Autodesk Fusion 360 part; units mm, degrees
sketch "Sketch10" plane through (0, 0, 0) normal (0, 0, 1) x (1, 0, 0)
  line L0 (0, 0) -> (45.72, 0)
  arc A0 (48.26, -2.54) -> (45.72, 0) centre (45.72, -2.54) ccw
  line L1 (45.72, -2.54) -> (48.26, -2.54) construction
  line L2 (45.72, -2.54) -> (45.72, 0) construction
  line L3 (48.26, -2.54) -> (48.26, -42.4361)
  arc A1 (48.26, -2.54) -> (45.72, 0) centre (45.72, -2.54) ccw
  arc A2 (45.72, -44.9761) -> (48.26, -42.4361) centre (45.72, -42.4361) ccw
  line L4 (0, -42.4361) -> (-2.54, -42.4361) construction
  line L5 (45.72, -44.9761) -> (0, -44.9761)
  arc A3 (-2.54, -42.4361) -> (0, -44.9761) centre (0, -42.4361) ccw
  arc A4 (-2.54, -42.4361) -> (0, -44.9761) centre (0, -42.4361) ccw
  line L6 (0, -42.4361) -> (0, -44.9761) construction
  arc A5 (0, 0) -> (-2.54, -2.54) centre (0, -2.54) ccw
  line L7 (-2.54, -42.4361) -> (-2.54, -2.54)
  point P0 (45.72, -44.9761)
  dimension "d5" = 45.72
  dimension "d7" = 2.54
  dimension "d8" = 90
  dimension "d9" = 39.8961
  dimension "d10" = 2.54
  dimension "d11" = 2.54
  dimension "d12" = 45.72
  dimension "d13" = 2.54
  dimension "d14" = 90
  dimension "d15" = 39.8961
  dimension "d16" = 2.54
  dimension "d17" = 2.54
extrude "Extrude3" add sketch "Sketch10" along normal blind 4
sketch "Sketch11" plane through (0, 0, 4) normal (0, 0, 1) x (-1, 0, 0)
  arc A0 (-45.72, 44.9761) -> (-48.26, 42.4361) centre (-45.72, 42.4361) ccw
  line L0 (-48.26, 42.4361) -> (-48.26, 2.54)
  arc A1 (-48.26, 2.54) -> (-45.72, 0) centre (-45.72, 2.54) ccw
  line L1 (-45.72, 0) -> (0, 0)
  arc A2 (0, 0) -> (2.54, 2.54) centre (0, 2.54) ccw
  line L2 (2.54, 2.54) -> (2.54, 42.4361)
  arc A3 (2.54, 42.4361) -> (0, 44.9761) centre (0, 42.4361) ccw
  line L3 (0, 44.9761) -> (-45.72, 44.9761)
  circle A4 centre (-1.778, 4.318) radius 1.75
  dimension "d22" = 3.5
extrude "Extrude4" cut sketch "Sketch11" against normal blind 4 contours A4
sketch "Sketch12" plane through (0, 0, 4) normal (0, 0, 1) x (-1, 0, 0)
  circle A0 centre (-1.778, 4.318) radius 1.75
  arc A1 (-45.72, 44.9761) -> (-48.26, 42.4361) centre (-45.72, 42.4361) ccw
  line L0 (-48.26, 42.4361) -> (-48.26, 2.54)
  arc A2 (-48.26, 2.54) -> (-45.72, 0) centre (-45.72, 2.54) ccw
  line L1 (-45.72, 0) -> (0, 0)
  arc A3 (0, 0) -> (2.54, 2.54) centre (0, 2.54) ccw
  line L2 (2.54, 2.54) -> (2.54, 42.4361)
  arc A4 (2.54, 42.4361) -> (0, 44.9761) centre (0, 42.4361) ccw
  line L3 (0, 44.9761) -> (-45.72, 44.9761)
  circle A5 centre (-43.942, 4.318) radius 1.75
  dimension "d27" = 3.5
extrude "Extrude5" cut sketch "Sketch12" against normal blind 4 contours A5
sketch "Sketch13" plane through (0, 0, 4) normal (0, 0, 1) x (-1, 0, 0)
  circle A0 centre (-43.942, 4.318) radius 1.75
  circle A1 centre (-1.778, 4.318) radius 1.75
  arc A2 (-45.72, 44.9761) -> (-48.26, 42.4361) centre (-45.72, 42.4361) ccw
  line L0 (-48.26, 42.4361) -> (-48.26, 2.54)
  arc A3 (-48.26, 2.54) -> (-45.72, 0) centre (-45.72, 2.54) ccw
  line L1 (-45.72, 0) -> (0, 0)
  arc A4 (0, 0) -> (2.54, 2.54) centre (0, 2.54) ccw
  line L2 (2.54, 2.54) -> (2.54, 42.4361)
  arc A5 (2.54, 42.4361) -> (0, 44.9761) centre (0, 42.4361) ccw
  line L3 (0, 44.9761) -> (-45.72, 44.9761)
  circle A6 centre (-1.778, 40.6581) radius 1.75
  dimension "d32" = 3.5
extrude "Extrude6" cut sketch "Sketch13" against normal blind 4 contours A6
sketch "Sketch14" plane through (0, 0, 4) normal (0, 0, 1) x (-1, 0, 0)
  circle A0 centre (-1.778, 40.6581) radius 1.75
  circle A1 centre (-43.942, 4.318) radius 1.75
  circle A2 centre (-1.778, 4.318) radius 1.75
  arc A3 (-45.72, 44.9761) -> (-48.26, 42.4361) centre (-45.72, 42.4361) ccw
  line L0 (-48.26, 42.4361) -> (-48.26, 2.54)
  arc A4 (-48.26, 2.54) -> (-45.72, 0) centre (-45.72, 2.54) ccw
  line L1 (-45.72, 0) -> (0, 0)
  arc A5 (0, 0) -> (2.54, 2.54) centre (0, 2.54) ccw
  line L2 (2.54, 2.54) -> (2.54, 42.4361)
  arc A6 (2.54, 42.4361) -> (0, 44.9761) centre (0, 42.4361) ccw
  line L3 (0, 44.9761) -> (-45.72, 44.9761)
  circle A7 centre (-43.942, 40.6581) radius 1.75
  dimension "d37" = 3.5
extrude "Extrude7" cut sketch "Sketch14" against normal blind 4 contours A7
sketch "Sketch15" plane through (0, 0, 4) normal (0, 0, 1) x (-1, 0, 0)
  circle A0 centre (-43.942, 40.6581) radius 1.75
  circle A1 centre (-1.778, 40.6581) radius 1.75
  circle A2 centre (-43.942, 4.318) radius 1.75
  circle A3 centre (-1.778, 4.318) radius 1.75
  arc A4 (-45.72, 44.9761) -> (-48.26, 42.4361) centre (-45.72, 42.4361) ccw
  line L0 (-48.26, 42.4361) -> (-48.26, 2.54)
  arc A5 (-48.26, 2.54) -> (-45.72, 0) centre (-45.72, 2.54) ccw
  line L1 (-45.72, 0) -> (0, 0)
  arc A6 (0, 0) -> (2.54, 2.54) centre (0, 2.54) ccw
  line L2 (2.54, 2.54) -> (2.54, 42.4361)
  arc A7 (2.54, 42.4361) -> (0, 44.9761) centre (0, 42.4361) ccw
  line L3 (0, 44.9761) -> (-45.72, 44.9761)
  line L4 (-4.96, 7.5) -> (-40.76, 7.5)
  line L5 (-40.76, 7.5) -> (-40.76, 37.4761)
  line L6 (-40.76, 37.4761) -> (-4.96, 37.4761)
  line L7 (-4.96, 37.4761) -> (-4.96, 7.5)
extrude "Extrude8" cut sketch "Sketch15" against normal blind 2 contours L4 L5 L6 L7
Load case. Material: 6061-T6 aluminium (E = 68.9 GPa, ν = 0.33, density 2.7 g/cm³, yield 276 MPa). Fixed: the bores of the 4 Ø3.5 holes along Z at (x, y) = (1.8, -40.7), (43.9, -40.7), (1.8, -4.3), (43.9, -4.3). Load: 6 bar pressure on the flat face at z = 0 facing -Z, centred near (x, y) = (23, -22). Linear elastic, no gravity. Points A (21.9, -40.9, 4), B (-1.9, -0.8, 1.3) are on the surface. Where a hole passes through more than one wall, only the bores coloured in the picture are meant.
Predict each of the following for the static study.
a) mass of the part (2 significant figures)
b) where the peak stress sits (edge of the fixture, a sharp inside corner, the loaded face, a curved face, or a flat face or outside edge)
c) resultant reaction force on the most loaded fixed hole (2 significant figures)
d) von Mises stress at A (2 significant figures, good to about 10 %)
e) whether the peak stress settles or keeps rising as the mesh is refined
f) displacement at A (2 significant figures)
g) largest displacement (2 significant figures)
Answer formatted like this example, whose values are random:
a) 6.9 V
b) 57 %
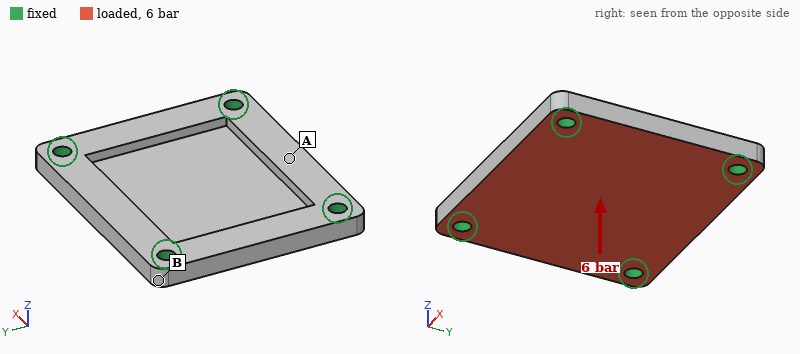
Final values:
a) 18 g
b) edge of the fixture
c) 380 N
d) 32 MPa
e) keeps rising
f) 24 µm
g) 61 µm
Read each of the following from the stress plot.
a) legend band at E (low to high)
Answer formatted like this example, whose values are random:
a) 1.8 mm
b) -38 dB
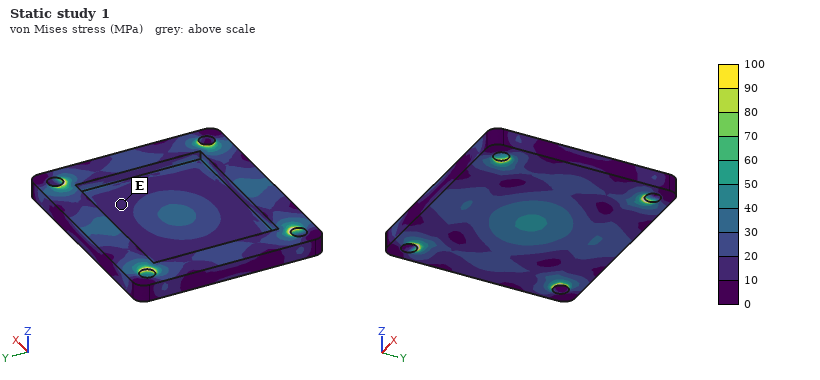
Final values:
a) 10 to 20 MPa
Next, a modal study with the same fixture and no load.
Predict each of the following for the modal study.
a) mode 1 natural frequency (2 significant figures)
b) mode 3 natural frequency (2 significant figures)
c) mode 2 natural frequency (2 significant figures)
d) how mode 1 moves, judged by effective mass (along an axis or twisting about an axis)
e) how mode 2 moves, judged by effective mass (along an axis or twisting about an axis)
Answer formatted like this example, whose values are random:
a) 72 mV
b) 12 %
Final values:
a) 8300 Hz
b) 14 kHz
c) 12 kHz
d) along Z
e) twisting about X
